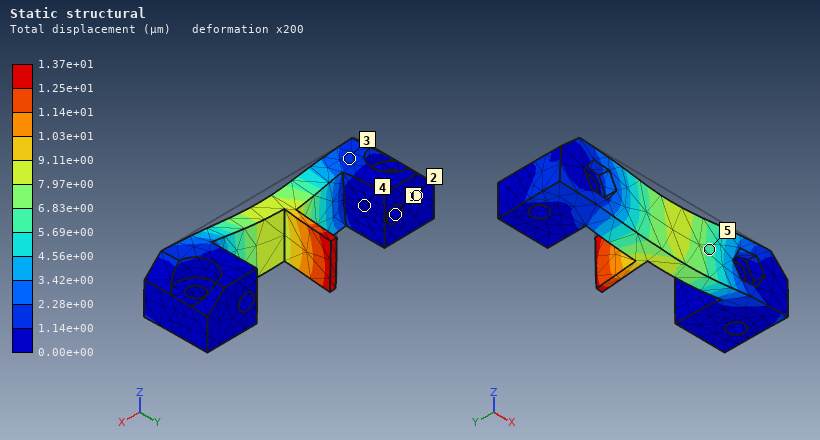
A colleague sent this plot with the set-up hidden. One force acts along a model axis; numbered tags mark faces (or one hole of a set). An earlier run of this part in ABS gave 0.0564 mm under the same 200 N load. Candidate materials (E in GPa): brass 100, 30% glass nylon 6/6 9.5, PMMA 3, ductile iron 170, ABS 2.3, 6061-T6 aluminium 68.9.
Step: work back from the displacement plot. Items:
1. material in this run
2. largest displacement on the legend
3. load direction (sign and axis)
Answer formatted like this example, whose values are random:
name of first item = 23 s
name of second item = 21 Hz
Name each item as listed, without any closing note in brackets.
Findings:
material in this run = 30% glass nylon 6/6
largest displacement on the legend = 1.37e+01 µm
load direction = -Z
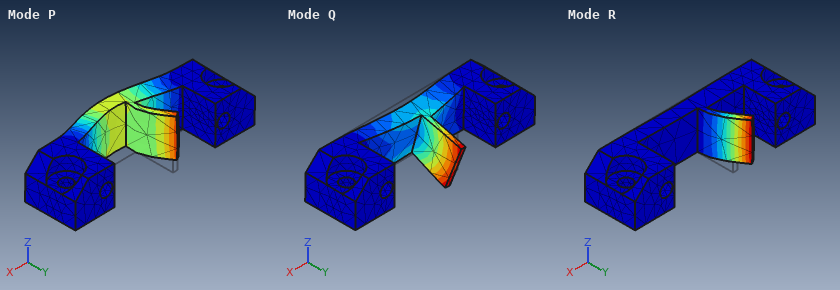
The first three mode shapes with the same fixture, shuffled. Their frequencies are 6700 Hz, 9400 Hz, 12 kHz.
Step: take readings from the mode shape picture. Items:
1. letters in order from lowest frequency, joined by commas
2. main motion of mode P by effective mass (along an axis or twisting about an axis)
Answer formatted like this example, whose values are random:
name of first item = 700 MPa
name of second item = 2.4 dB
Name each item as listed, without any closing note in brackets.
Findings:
letters in order from lowest frequency, joined by commas = R, P, Q
main motion of mode P by effective mass = along Y
